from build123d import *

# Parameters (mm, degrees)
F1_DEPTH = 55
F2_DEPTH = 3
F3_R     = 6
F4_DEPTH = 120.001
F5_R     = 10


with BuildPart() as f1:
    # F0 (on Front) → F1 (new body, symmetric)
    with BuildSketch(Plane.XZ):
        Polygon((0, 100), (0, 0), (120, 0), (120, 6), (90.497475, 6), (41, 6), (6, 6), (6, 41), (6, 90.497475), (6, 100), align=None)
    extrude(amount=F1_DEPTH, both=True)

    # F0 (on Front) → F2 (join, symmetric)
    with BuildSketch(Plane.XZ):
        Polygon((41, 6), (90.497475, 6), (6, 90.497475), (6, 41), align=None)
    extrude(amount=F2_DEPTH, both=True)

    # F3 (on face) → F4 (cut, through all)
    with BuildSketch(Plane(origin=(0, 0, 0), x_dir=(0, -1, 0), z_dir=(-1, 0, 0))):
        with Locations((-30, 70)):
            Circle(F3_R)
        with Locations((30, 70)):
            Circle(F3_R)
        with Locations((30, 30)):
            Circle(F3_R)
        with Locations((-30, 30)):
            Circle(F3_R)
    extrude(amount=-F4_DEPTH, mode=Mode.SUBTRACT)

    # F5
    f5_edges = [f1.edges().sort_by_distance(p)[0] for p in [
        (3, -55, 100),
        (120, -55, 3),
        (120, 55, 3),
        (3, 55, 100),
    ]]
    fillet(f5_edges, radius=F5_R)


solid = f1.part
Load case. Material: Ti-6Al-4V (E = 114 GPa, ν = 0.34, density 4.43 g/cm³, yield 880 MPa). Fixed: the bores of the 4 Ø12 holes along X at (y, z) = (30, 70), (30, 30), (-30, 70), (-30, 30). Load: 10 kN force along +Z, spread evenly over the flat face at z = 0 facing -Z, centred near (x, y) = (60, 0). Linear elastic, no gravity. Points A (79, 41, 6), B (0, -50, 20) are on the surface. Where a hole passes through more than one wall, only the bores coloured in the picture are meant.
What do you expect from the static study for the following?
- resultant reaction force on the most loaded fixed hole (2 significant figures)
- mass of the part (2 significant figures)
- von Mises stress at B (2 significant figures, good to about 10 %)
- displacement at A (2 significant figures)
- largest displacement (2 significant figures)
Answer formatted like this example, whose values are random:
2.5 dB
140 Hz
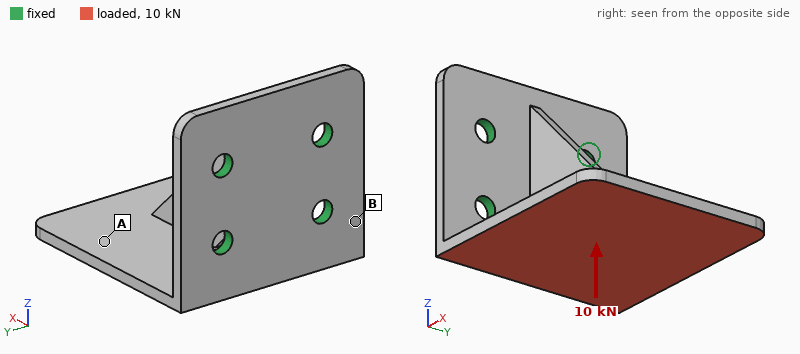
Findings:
5.4 kN
690 g
110 MPa
0.59 mm
0.98 mm
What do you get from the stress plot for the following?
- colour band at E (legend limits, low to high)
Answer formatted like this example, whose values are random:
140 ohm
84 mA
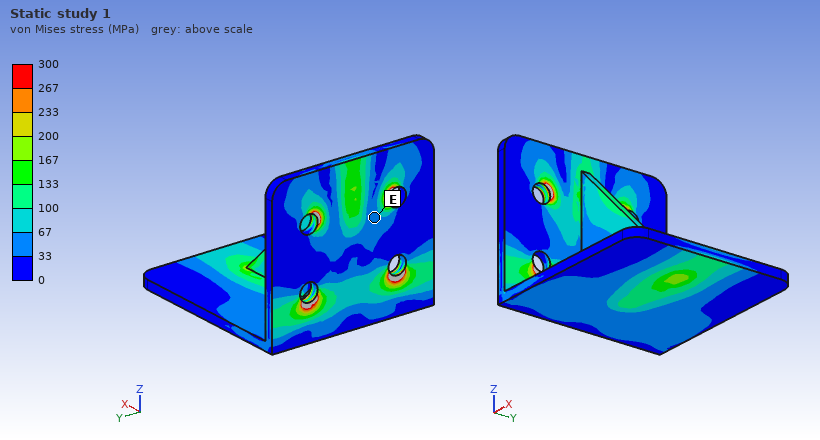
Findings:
33 to 67 MPa
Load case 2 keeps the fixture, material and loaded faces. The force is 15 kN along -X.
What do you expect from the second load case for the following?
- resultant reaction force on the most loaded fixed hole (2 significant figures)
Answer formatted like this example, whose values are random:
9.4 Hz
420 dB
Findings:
9.7 kN
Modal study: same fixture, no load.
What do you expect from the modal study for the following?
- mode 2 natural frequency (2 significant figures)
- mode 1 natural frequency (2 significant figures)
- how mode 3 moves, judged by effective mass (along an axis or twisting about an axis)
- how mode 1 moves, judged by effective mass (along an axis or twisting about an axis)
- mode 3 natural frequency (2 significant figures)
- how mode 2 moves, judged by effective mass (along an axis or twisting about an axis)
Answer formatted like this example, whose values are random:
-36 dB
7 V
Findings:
1100 Hz
860 Hz
along Y
along Y
1100 Hz
along Z
